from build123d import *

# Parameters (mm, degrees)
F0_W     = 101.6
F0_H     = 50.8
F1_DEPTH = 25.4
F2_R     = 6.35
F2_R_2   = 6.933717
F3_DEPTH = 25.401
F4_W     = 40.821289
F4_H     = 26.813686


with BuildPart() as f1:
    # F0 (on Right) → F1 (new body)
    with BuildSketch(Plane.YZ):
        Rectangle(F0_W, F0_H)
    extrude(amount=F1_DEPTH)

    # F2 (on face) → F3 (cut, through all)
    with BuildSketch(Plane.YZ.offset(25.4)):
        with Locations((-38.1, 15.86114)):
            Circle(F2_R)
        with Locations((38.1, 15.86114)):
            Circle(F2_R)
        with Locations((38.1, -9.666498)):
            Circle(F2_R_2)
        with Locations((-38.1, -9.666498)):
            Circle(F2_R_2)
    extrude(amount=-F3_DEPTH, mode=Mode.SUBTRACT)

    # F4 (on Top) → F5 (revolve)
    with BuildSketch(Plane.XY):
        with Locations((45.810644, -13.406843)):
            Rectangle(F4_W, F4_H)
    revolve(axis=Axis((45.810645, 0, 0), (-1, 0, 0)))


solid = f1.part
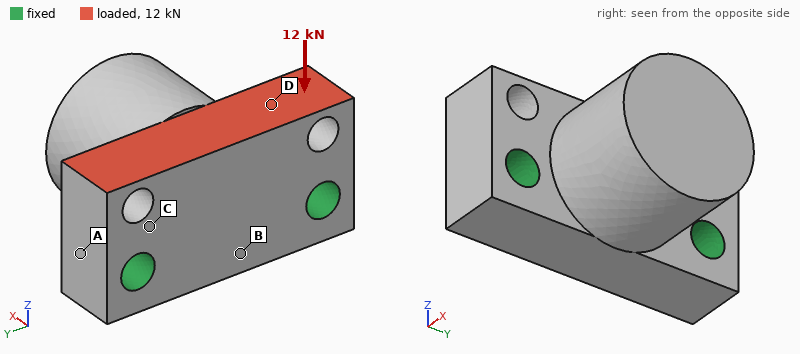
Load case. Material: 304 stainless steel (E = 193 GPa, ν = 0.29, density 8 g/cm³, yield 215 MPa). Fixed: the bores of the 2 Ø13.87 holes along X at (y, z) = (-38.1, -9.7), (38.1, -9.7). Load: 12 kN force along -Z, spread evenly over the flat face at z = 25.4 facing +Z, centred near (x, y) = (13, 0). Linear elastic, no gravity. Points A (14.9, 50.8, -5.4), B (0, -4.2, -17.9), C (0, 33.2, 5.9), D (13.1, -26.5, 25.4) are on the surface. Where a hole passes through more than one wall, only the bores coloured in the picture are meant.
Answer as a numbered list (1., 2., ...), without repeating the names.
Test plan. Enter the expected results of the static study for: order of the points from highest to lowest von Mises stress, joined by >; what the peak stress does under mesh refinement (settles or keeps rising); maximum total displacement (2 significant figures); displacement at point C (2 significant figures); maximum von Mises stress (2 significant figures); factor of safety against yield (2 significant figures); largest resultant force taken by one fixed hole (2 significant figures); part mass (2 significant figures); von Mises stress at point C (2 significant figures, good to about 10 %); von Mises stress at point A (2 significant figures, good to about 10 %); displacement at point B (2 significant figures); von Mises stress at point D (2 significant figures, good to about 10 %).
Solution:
1. C > D > A > B
2. settles
3. 2.4 µm
4. 0.49 µm
5. 26 MPa
6. 8.2
7. 6.1 kN
8. 1.7 kg
9. 12 MPa
10. 4.3 MPa
11. 1.2 µm
12. 8.3 MPa
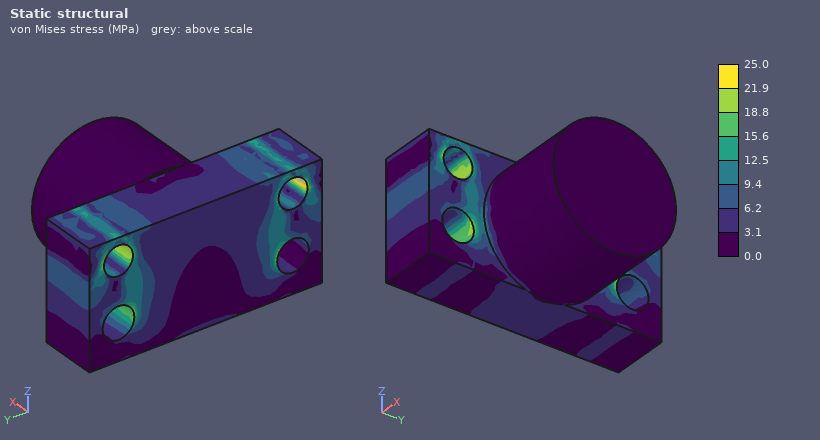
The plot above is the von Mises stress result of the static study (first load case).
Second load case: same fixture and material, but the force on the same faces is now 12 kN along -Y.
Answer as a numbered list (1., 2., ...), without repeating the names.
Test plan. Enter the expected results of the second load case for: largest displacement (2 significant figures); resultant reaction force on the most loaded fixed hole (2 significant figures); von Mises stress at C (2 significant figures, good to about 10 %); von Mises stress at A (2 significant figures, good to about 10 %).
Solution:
1. 5.2 µm
2. 7.8 kN
3. 11 MPa
4. 9.4 MPa
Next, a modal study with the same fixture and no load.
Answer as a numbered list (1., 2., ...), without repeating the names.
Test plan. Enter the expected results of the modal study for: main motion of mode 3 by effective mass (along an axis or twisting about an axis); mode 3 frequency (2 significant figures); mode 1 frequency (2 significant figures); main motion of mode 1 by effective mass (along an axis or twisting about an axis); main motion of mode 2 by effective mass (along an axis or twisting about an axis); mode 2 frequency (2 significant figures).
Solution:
1. along X
2. 9900 Hz
3. 4300 Hz
4. along Z
5. along Y
6. 8400 Hz
